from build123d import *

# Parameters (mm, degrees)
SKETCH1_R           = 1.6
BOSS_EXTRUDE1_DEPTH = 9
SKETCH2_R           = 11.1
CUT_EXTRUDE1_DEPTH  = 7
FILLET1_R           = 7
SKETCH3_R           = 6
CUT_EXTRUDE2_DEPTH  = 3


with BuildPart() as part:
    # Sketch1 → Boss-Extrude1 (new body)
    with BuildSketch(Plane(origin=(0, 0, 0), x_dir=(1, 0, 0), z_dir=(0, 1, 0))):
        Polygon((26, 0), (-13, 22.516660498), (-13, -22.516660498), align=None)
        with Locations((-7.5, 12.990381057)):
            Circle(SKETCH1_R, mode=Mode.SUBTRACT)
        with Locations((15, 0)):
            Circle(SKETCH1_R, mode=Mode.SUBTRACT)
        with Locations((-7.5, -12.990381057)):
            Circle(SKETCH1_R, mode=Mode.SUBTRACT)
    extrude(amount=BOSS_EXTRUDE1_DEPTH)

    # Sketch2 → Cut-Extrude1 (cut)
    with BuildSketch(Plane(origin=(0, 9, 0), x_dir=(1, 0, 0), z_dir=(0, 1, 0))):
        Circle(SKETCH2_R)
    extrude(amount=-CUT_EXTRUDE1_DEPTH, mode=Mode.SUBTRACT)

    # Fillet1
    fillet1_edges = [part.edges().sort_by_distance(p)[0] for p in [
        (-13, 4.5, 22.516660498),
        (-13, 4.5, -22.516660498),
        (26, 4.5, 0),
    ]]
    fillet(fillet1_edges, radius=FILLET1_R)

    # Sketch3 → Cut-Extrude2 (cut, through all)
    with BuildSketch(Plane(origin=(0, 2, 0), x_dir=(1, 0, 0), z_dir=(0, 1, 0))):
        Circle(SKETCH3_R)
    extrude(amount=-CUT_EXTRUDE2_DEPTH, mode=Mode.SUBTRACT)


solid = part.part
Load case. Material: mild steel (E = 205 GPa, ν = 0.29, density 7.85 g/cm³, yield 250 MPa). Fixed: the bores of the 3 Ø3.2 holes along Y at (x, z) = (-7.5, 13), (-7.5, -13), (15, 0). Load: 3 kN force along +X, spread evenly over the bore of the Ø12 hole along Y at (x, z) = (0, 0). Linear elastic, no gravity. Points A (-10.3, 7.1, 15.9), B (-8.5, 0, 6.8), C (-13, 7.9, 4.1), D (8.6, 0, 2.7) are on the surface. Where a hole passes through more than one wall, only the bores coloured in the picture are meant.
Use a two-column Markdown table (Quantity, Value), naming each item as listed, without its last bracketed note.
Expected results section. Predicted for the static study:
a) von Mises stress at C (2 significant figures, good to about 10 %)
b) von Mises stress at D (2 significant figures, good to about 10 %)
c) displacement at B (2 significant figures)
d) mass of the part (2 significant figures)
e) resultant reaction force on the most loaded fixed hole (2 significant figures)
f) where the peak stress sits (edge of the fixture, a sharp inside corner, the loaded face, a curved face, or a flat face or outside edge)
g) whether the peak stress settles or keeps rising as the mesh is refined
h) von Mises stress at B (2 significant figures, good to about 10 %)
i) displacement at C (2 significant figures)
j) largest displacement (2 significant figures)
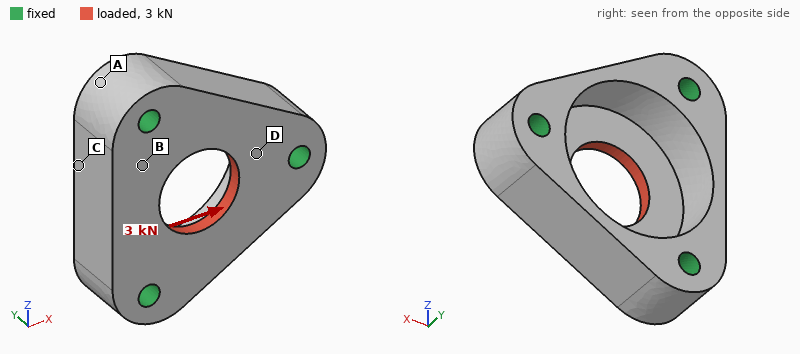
| Quantity | Value |
|---|---|
| von Mises stress at C | 14 MPa |
| von Mises stress at D | 54 MPa |
| displacement at B | 2.4 µm |
| mass of the part | 30 g |
| resultant reaction force on the most loaded fixed hole | 1.0 kN |
| where the peak stress sits | edge of the fixture |
| whether the peak stress settles or keeps rising as the mesh is refined | keeps rising |
| von Mises stress at B | 47 MPa |
| displacement at C | 0.89 µm |
| largest displacement | 5.3 µm |
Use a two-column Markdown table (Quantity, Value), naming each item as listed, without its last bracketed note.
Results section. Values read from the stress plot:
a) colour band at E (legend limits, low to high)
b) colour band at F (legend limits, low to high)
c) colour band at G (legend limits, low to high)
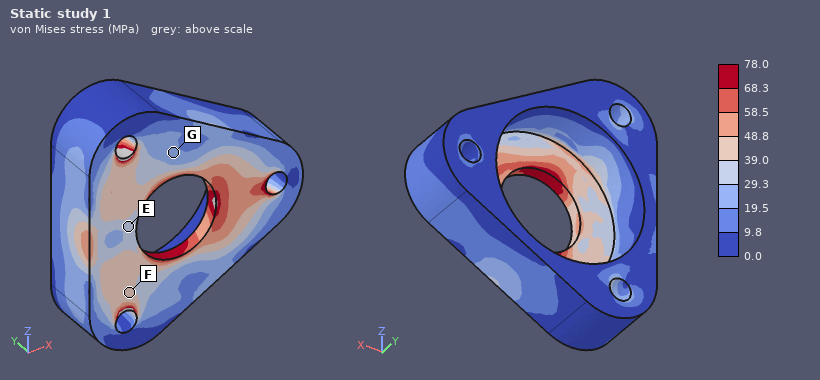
| Quantity | Value |
|---|---|
| colour band at E | 29.3 to 39.0 MPa |
| colour band at F | 39.0 to 48.8 MPa |
| colour band at G | 19.5 to 29.3 MPa |
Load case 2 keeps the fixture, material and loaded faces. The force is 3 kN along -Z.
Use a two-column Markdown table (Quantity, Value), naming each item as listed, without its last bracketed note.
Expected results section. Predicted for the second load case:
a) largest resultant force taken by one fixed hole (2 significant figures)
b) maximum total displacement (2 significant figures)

| Quantity | Value |
|---|---|
| largest resultant force taken by one fixed hole | 1.1 kN |
| maximum total displacement | 4.7 µm |
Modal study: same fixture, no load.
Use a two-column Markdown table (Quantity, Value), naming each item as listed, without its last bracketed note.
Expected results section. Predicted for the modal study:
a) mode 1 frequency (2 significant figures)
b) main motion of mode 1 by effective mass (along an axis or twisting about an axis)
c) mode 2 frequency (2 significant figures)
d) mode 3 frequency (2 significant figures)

| Quantity | Value |
|---|---|
| mode 1 frequency | 42 kHz |
| main motion of mode 1 by effective mass | along Y |
| mode 2 frequency | 48 kHz |
| mode 3 frequency | 48 kHz |
